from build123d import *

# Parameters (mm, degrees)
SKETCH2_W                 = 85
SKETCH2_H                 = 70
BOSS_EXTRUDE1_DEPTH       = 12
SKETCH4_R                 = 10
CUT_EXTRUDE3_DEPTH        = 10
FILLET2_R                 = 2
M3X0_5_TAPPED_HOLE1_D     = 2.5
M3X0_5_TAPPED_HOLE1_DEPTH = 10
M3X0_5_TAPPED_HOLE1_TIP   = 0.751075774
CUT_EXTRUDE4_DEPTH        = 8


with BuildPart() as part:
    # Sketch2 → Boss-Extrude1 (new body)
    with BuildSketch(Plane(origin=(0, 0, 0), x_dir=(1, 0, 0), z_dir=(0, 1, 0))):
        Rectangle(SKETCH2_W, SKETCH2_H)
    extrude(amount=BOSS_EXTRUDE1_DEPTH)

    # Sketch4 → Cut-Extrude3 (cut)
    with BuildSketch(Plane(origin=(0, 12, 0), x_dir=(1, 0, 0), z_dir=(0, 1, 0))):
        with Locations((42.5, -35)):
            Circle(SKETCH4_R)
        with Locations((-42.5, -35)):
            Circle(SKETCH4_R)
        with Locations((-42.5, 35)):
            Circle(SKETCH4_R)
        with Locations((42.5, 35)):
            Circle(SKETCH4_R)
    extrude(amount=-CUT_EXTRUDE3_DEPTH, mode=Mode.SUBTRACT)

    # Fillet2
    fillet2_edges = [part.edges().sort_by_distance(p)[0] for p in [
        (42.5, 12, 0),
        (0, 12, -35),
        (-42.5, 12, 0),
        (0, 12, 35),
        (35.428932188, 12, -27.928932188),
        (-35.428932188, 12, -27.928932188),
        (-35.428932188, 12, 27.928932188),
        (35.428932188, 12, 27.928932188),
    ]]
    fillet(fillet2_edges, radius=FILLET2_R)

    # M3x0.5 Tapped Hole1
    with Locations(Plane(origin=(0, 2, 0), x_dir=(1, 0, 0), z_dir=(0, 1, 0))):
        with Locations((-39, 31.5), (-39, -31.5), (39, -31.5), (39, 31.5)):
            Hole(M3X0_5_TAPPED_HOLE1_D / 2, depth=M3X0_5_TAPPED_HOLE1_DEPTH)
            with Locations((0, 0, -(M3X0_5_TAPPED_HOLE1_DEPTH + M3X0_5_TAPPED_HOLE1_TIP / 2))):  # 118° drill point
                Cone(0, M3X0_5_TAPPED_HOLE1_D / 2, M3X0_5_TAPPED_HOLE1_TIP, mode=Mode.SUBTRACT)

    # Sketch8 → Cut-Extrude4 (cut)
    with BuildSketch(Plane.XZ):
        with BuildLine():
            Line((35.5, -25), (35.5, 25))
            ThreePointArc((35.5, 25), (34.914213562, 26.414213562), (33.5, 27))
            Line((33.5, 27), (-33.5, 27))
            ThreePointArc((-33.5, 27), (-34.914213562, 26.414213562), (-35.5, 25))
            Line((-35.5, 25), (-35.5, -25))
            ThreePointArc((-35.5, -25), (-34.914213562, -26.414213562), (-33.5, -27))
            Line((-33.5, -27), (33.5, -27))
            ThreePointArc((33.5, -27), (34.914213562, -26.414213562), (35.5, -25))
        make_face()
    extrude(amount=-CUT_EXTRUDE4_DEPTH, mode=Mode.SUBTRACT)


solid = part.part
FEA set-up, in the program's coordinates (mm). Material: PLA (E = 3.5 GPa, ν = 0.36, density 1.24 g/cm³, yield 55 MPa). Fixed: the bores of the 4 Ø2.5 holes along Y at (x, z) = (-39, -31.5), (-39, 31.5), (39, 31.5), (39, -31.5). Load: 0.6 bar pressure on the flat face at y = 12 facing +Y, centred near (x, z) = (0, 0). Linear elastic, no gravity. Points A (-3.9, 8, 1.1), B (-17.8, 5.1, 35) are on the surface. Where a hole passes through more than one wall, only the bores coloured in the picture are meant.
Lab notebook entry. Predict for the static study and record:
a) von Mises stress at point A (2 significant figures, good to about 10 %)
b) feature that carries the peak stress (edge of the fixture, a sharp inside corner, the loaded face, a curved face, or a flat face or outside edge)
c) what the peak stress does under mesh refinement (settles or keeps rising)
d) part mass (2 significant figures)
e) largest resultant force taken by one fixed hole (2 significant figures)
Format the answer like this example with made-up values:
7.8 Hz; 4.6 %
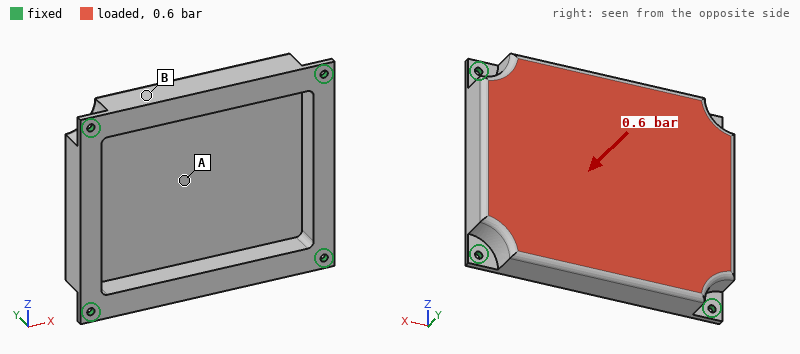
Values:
2.8 MPa; edge of the fixture; keeps rising; 46 g; 130 N
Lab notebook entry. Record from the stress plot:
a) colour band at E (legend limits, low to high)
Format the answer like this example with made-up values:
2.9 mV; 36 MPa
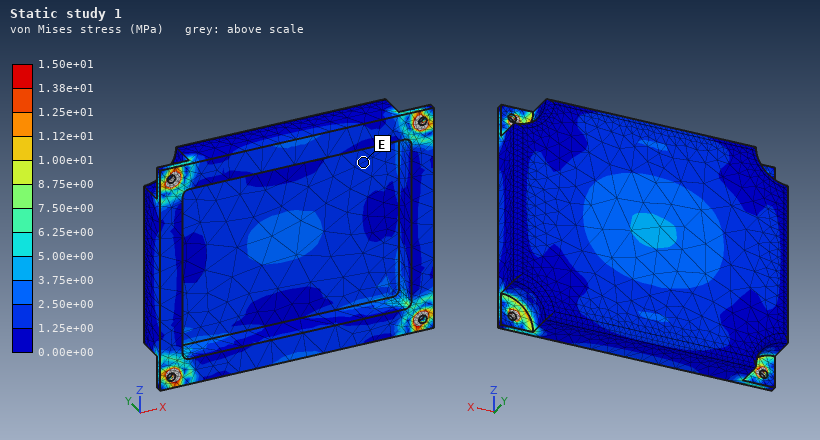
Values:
1.25e+00 to 2.50e+00 MPa
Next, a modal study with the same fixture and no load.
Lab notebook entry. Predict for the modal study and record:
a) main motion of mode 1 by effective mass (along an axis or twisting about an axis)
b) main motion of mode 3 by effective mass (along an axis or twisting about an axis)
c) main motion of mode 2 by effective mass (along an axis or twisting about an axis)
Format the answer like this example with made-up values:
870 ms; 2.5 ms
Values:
along Y; twisting about Z; twisting about X
